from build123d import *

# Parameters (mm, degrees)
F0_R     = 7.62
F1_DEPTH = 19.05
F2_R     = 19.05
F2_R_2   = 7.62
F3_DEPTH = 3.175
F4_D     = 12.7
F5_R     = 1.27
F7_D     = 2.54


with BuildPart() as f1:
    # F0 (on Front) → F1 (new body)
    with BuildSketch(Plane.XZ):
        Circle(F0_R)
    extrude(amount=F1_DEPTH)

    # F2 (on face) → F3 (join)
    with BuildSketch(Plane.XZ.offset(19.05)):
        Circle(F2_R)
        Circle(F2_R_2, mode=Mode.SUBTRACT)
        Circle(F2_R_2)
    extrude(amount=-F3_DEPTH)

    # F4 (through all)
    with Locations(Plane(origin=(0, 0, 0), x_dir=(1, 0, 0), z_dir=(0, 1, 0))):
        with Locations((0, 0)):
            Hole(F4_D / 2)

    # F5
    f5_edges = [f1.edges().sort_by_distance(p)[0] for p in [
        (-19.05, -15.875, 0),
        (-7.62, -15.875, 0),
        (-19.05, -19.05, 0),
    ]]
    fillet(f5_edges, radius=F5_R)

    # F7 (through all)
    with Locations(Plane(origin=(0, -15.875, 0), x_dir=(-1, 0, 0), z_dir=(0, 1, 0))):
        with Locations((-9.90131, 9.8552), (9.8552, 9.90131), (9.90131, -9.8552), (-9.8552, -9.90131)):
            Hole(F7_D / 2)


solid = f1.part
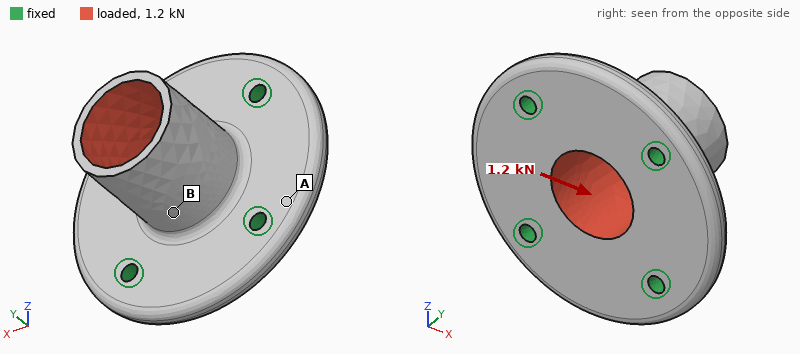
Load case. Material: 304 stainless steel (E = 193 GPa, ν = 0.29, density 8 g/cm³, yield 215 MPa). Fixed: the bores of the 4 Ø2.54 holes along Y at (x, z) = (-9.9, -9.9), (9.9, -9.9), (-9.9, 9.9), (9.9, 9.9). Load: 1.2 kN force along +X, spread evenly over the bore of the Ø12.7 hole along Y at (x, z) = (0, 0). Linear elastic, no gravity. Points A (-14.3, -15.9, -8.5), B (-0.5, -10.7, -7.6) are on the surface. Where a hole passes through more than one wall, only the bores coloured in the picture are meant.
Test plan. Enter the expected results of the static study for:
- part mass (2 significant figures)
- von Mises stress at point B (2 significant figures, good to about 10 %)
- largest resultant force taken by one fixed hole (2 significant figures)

32 g
35 MPa
410 N
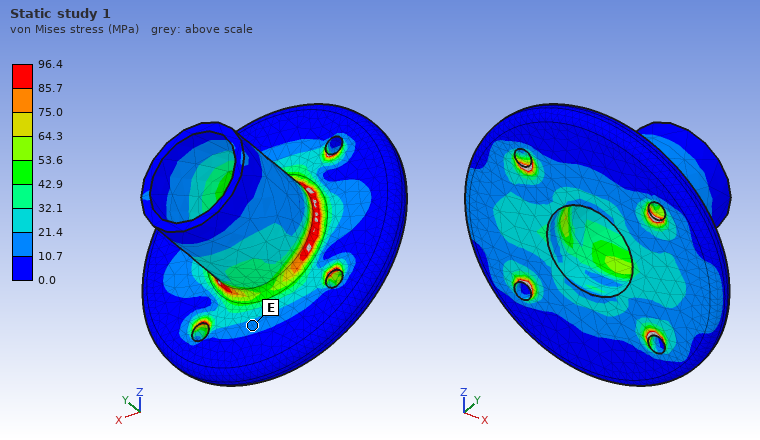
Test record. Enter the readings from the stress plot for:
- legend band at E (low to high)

10.7 to 21.4 MPa
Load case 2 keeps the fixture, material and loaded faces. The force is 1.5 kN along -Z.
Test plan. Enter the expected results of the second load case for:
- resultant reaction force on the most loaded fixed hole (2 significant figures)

520 N
